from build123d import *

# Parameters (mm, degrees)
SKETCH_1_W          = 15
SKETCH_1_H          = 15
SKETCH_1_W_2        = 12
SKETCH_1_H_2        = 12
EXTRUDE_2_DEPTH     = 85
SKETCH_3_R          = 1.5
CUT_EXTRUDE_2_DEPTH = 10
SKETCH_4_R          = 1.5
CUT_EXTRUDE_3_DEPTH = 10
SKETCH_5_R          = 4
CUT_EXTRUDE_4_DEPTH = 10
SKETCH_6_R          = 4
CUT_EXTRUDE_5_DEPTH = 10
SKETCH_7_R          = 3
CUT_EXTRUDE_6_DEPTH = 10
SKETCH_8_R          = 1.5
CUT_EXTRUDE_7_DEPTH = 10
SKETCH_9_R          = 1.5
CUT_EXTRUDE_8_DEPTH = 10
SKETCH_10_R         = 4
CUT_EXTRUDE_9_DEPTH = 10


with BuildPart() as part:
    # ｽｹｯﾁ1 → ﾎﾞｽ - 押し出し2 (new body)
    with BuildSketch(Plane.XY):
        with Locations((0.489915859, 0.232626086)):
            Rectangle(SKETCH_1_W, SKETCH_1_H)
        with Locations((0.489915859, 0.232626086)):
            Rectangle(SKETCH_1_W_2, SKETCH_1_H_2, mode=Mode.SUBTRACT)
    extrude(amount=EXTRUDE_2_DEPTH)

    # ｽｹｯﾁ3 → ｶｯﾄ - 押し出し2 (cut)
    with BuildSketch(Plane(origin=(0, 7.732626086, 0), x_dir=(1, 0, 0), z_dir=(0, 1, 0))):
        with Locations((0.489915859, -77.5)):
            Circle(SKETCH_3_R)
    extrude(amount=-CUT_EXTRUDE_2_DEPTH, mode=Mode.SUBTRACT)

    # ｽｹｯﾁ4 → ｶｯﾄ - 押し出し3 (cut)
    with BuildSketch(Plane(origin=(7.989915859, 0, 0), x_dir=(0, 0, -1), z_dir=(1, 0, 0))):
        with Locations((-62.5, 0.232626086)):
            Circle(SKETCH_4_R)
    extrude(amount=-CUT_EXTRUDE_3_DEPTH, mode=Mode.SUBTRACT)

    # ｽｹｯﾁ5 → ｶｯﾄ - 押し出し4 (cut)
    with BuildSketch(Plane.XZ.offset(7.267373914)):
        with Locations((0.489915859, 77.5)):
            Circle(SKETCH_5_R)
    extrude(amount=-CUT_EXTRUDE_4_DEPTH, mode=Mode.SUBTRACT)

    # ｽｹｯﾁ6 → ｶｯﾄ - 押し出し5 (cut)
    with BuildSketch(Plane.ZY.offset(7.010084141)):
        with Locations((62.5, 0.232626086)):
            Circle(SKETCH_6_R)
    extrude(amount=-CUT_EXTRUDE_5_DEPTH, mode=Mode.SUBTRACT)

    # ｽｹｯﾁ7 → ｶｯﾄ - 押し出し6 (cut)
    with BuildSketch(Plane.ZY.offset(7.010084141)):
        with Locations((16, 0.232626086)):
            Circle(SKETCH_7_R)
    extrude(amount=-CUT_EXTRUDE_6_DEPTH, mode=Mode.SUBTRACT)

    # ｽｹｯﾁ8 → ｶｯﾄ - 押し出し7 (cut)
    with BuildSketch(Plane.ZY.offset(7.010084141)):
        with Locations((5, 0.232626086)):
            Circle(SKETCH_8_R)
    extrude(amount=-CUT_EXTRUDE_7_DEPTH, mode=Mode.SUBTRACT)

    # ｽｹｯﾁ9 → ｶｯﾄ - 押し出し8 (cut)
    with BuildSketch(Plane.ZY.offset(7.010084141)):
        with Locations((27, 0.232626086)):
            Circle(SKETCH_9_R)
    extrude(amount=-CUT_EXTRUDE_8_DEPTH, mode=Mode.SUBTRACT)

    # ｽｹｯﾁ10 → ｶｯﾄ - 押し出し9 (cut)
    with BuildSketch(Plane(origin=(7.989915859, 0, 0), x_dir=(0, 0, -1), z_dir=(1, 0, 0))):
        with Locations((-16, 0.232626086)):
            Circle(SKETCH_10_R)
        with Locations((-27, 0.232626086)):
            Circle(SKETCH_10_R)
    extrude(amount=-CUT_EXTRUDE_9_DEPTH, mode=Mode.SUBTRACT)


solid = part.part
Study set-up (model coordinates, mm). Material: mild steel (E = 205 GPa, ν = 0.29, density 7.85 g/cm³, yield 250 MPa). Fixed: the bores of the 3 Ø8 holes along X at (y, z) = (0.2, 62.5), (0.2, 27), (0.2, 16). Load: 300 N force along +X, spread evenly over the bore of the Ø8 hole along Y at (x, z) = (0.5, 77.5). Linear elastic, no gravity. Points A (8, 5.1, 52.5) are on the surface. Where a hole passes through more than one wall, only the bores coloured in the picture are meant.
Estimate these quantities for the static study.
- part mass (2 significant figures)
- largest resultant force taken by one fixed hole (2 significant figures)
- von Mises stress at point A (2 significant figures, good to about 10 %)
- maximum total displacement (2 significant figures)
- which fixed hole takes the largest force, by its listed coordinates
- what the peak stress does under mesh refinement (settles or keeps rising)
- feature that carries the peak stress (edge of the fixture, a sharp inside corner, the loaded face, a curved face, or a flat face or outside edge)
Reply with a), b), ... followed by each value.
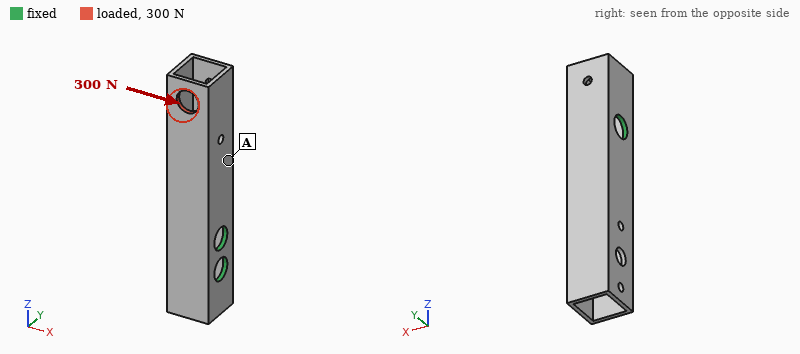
a) 51 g
b) 420 N
c) 9.2 MPa
d) 13 µm
e) (0.2, 62.5)
f) keeps rising
g) edge of the fixture
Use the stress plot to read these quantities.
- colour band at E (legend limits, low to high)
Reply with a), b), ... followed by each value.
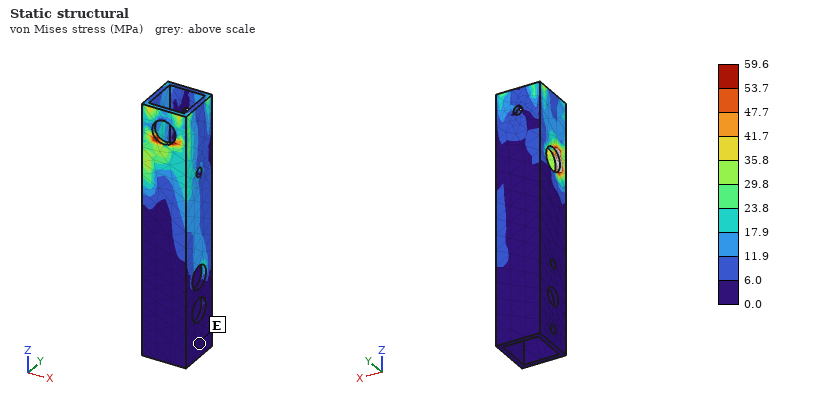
a) 0.0 to 6.0 MPa
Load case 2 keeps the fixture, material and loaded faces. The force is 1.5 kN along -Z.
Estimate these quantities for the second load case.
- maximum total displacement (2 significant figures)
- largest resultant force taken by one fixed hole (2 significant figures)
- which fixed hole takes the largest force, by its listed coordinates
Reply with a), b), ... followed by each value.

a) 20 µm
b) 950 N
c) (0.2, 62.5)
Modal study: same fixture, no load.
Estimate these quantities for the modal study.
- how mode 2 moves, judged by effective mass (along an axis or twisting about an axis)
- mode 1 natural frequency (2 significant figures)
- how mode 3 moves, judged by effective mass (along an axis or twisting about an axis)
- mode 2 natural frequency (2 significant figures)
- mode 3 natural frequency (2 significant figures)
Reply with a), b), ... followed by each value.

a) along Y
b) 6100 Hz
c) along X
d) 9400 Hz
e) 11 kHz
